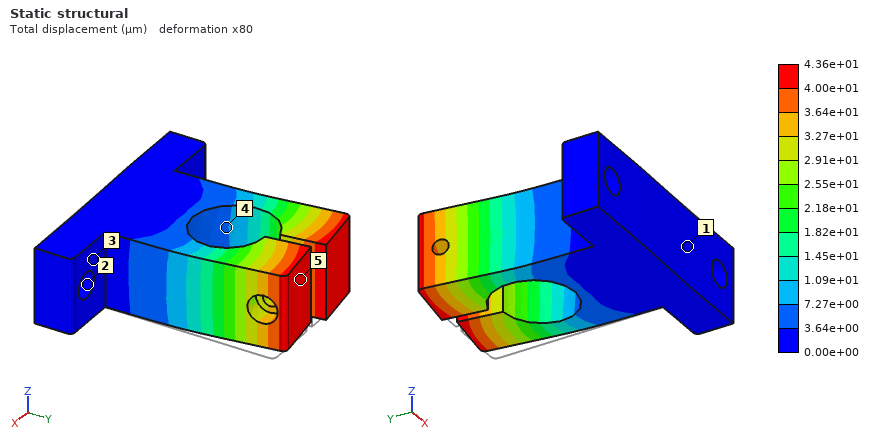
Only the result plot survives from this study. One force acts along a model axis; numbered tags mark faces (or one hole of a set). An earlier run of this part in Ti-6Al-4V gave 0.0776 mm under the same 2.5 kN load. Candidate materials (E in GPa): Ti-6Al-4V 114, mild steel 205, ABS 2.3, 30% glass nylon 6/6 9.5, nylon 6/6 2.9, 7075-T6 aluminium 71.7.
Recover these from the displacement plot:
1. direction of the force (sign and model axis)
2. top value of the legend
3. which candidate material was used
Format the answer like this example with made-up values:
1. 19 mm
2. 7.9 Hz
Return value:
1. -X
2. 4.36e+01 µm
3. mild steel
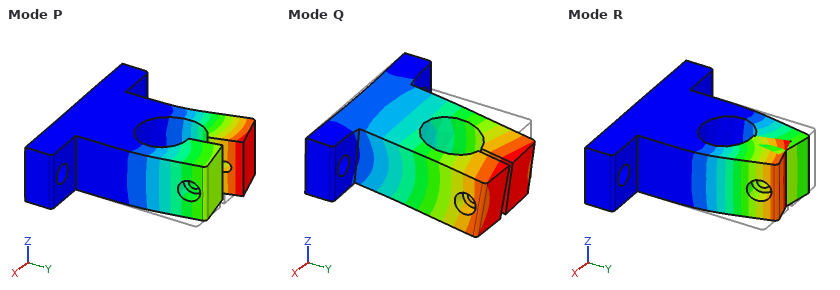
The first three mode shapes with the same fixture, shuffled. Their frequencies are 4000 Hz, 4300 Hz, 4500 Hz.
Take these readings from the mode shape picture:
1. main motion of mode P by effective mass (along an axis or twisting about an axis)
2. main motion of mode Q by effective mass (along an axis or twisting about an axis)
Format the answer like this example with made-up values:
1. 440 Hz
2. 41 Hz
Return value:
1. along X
2. along Z
